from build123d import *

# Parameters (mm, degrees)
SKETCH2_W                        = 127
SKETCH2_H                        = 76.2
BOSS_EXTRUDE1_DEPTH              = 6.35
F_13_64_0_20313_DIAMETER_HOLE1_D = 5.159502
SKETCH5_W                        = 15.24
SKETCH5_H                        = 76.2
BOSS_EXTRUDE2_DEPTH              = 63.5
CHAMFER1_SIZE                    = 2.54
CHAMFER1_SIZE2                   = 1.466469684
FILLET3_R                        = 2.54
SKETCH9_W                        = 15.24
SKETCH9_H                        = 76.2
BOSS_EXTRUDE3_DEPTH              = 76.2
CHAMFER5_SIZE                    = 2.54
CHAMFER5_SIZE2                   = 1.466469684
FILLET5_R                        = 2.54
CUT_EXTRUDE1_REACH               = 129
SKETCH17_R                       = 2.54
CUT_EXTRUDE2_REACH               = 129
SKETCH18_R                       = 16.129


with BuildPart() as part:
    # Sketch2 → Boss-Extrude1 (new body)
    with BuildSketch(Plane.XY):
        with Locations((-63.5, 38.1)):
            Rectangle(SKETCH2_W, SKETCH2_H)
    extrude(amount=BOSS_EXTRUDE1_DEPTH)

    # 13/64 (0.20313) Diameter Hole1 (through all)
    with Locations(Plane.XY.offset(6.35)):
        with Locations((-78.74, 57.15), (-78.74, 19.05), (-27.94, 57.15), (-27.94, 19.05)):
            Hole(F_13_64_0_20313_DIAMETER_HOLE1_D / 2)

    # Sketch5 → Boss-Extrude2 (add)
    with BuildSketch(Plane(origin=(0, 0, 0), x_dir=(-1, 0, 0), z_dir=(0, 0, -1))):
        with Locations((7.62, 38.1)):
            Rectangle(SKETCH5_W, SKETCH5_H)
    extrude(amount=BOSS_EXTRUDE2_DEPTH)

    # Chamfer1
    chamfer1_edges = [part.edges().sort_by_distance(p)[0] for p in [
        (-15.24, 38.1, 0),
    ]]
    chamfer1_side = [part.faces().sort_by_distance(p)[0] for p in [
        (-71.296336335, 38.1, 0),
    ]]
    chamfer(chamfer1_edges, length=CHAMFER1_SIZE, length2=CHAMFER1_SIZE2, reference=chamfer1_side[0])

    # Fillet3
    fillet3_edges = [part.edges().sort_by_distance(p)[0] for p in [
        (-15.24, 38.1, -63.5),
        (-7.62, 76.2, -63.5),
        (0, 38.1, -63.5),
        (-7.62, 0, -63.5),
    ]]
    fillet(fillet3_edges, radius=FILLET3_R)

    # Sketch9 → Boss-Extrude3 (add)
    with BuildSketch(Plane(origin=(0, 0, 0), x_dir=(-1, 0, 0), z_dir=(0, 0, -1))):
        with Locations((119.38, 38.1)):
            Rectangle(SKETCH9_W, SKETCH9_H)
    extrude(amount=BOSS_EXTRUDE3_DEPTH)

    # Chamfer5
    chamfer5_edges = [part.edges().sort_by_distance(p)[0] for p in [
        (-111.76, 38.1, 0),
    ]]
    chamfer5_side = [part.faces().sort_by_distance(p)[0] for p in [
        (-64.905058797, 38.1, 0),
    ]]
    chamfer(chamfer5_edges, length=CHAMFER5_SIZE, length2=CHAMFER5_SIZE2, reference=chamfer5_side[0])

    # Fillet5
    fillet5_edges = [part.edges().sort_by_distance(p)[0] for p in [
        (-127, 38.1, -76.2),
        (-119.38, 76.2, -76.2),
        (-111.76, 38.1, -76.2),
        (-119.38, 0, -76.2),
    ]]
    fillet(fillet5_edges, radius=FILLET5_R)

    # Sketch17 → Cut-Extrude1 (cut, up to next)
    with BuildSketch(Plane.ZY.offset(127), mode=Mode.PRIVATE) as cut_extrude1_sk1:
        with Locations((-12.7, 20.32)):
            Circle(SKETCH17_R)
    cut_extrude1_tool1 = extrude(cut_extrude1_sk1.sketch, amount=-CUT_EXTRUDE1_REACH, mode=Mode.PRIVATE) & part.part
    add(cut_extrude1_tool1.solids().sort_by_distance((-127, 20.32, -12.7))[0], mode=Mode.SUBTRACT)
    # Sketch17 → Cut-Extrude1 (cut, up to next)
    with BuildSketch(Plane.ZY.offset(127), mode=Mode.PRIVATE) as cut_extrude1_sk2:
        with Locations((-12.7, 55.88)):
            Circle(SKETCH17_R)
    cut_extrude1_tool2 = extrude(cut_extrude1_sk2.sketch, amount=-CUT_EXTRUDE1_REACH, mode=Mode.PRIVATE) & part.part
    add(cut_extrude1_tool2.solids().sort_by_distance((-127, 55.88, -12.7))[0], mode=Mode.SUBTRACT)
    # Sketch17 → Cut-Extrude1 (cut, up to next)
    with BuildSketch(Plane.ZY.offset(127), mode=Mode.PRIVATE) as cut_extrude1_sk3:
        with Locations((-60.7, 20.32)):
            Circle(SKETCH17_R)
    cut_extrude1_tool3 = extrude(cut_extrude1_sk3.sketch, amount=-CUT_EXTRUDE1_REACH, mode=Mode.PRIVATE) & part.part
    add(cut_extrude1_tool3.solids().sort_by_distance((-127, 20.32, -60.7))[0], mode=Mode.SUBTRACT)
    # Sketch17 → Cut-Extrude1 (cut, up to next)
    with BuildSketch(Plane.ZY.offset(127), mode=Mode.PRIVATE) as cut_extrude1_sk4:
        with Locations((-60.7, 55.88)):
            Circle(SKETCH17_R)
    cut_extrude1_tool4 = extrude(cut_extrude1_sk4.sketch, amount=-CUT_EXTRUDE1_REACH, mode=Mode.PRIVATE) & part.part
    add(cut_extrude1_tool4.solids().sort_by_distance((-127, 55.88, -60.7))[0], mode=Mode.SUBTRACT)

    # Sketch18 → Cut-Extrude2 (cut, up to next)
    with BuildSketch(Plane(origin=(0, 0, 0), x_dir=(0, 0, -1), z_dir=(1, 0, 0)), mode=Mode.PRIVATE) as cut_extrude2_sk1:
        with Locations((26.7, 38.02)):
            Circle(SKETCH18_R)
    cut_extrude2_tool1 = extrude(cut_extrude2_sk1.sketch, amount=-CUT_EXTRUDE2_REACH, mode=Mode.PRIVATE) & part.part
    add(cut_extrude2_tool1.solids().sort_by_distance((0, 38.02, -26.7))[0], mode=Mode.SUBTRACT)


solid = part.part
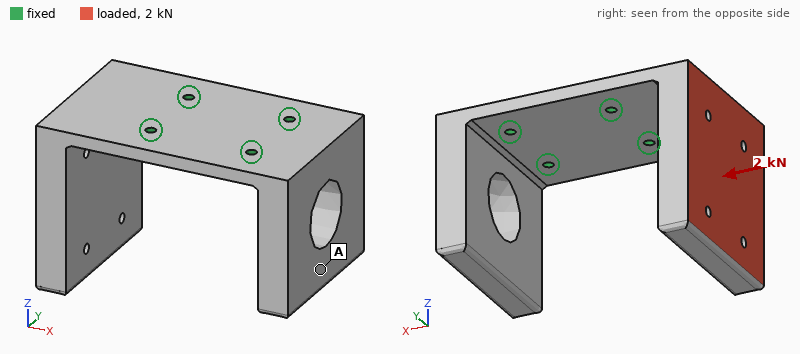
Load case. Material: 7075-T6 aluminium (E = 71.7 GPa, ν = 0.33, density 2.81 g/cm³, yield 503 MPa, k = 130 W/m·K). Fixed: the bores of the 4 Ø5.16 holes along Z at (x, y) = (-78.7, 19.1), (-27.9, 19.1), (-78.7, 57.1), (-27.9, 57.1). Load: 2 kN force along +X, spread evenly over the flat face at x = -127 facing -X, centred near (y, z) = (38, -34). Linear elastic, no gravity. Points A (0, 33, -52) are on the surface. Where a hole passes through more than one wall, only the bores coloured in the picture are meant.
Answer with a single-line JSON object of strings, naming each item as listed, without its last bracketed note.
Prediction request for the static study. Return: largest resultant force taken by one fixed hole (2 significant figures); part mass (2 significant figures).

{"largest resultant force taken by one fixed hole": "890 N", "part mass": "590 g"}
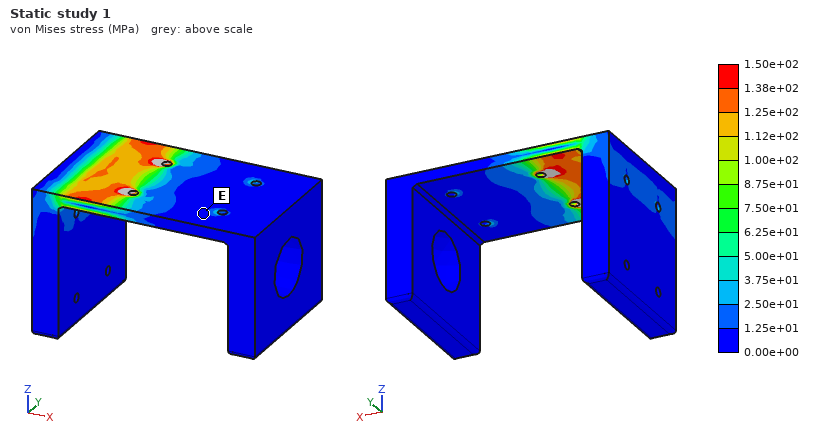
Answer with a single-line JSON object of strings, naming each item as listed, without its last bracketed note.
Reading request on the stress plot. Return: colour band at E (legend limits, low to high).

{"colour band at E": "0.00e+00 to 1.25e+01 MPa"}
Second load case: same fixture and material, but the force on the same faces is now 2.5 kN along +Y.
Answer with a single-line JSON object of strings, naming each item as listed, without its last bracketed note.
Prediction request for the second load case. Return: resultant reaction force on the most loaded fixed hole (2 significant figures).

{"resultant reaction force on the most loaded fixed hole": "3.2 kN"}
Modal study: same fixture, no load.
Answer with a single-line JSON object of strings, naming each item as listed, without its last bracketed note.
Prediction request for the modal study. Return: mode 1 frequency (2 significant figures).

{"mode 1 frequency": "350 Hz"}
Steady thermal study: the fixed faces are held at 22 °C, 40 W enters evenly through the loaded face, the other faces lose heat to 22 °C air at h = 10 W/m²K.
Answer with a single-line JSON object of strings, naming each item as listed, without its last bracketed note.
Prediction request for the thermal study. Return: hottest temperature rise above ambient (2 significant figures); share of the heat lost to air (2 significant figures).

{"hottest temperature rise above ambient": "32 K", "share of the heat lost to air": "10 %"}
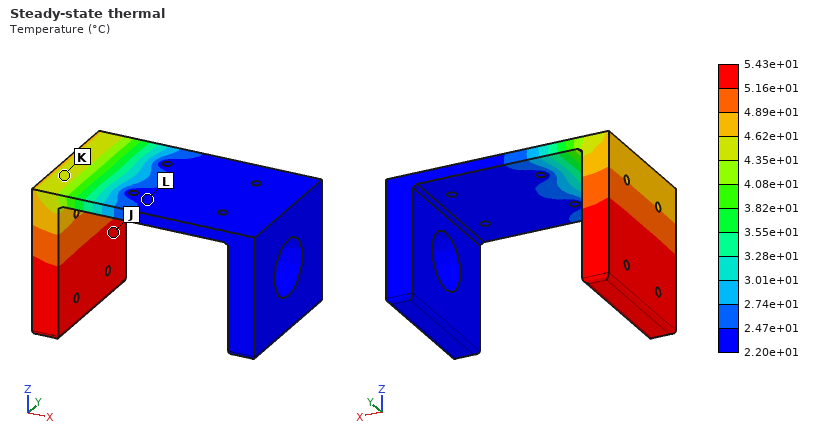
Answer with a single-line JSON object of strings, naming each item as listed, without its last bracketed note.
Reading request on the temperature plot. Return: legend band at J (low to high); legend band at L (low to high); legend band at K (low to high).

{"legend band at J": "5.16e+01 to 5.43e+01 °C", "legend band at L": "2.20e+01 to 2.47e+01 °C", "legend band at K": "4.35e+01 to 4.62e+01 °C"}
